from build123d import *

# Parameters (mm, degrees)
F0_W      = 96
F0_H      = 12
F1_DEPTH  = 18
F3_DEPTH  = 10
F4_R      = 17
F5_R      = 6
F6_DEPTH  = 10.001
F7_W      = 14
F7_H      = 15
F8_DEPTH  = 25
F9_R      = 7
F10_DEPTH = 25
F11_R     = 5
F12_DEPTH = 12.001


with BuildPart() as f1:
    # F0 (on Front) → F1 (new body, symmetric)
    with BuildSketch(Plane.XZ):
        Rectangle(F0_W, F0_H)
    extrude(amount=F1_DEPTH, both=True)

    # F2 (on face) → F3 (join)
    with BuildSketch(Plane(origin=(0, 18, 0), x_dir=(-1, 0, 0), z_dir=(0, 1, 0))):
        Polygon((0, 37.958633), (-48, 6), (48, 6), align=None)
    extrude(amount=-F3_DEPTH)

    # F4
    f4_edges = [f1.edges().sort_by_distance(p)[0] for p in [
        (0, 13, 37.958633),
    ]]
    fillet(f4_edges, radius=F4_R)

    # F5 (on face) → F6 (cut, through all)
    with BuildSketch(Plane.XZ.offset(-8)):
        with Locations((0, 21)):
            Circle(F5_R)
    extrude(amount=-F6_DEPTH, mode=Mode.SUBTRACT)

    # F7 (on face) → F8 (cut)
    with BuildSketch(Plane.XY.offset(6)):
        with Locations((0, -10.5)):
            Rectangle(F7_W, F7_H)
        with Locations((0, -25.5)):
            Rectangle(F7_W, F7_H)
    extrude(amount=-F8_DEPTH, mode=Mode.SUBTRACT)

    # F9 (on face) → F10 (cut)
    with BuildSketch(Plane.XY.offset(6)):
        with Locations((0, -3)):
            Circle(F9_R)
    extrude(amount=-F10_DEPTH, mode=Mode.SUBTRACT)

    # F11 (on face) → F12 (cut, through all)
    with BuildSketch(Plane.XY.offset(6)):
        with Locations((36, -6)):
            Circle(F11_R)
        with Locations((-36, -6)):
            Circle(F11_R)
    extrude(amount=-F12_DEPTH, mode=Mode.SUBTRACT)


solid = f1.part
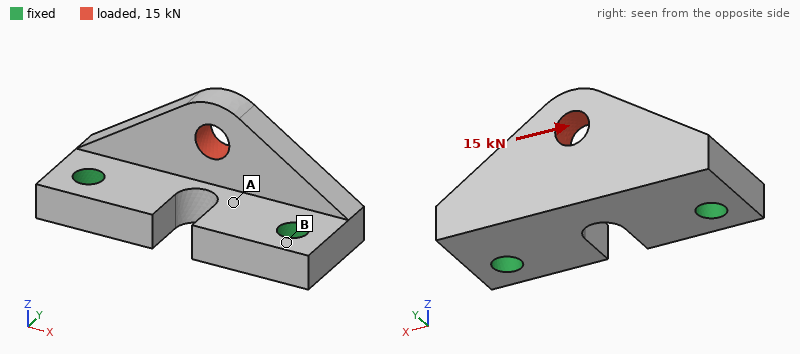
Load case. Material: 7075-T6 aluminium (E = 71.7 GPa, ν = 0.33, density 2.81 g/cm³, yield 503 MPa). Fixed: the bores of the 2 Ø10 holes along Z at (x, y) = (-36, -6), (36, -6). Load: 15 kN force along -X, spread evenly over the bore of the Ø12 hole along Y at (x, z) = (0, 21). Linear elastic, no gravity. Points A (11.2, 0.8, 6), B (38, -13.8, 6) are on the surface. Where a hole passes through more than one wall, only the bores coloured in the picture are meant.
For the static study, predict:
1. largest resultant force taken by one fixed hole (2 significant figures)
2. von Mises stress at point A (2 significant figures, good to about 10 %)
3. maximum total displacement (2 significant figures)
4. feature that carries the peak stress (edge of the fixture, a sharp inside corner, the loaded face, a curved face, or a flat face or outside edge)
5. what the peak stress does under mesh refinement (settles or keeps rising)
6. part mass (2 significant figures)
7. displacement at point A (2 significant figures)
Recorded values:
9.1 kN
45 MPa
66 µm
edge of the fixture
keeps rising
140 g
14 µm
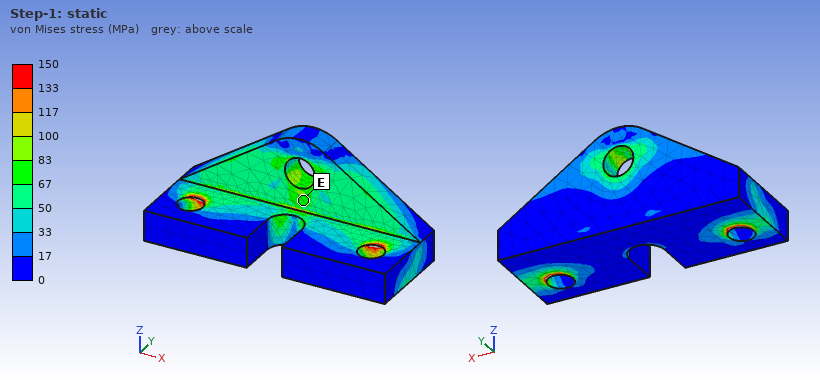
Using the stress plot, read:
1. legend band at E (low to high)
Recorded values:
67 to 83 MPa
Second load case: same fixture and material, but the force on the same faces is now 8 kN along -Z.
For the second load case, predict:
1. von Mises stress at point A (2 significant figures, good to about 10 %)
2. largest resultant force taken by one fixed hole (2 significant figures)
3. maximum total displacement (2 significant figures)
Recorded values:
19 MPa
4.1 kN
0.10 mm
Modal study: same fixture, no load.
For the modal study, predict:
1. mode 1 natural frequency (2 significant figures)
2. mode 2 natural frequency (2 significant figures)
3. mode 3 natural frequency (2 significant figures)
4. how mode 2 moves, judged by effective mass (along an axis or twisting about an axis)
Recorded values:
5900 Hz
11 kHz
12 kHz
along Z
